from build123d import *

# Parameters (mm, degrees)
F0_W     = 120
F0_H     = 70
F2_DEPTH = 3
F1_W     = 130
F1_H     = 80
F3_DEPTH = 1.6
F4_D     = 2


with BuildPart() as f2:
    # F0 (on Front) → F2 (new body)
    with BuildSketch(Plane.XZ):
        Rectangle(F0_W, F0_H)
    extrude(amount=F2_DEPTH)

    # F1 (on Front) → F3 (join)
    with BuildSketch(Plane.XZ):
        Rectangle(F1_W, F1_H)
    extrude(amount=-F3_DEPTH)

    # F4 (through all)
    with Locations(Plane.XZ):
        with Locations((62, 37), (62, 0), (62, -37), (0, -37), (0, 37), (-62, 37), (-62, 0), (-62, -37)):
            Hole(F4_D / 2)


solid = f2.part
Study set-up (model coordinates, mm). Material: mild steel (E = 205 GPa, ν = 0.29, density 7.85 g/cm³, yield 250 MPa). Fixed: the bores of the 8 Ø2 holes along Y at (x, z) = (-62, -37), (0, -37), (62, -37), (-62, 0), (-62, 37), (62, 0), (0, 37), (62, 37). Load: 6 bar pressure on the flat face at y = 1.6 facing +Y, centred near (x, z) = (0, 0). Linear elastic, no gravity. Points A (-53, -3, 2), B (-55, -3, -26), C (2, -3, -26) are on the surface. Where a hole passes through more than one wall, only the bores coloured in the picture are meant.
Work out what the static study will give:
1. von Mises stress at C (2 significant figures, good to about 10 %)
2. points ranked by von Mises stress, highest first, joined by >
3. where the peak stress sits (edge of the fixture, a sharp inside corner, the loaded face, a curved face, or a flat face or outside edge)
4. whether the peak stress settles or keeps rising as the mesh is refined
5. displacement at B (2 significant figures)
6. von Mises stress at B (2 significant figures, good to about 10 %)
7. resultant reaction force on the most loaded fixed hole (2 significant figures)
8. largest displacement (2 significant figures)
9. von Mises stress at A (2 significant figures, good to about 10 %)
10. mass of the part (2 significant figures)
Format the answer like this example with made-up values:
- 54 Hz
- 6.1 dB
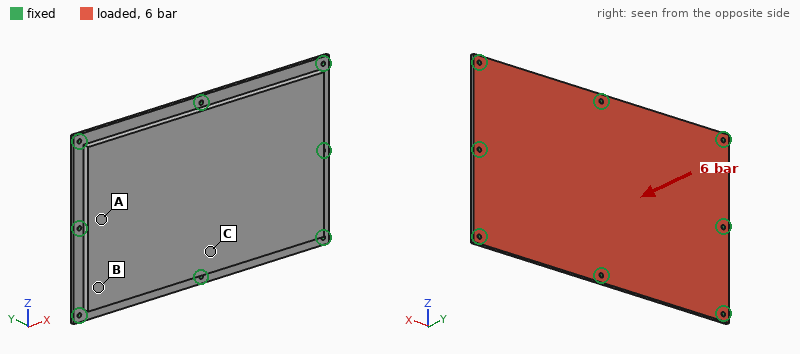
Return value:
- 93 MPa
- C > A > B
- edge of the fixture
- keeps rising
- 25 µm
- 25 MPa
- 2.8 kN
- 88 µm
- 48 MPa
- 330 g
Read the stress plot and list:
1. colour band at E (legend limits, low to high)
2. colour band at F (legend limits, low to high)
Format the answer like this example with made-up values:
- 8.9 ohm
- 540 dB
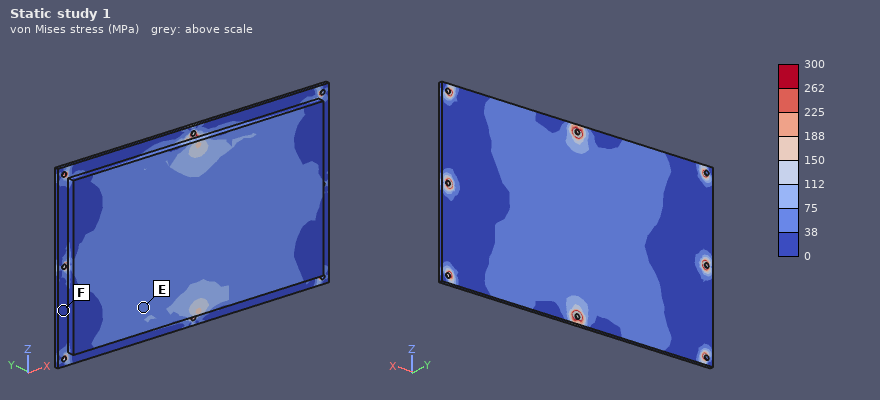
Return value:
- 38 to 75 MPa
- 0 to 38 MPa
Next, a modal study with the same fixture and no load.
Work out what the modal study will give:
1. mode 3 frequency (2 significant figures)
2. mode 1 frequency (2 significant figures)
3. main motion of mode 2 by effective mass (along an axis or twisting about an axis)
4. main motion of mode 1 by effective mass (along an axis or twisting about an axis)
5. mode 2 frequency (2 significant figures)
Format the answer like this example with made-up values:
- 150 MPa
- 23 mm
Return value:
- 4400 Hz
- 2600 Hz
- twisting about Z
- along Y
- 3200 Hz
